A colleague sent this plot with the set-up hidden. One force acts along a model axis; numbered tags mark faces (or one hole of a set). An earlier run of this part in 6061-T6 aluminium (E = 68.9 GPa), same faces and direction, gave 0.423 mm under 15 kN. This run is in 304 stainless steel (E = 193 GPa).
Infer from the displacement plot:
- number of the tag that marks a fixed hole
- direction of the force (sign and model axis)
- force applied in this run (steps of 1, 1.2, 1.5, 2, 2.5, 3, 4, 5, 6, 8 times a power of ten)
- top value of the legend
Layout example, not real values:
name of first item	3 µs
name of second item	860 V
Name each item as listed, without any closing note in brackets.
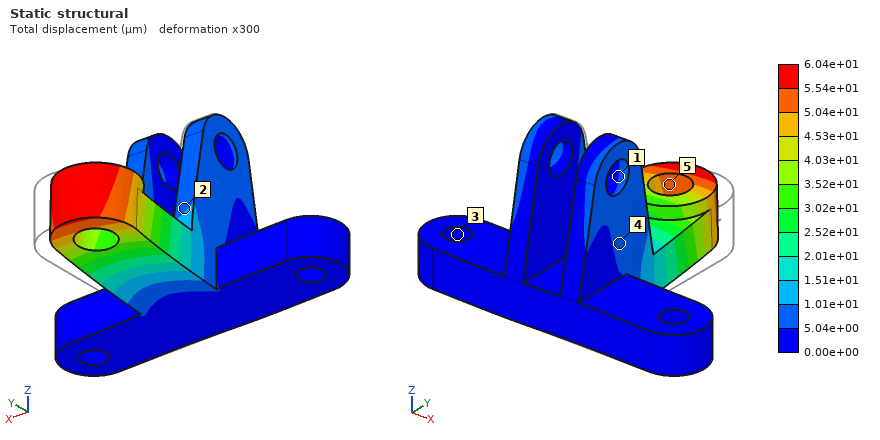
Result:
number of the tag that marks a fixed hole	3
direction of the force	-X
force applied in this run	6 kN
top value of the legend	6.04e+01 µm
